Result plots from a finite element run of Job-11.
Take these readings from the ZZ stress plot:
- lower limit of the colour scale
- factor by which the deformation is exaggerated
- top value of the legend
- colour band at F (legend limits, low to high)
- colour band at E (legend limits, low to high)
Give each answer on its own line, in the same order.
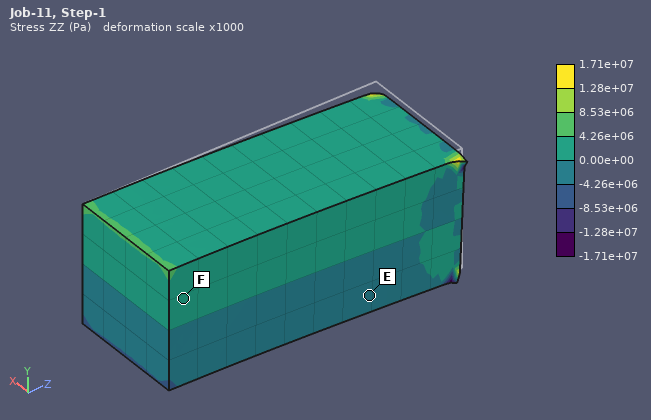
-1.71e+07 Pa
1000
1.71e+07 Pa
0.00e+00 to 4.26e+06 Pa
-4.26e+06 to 0.00e+00 Pa
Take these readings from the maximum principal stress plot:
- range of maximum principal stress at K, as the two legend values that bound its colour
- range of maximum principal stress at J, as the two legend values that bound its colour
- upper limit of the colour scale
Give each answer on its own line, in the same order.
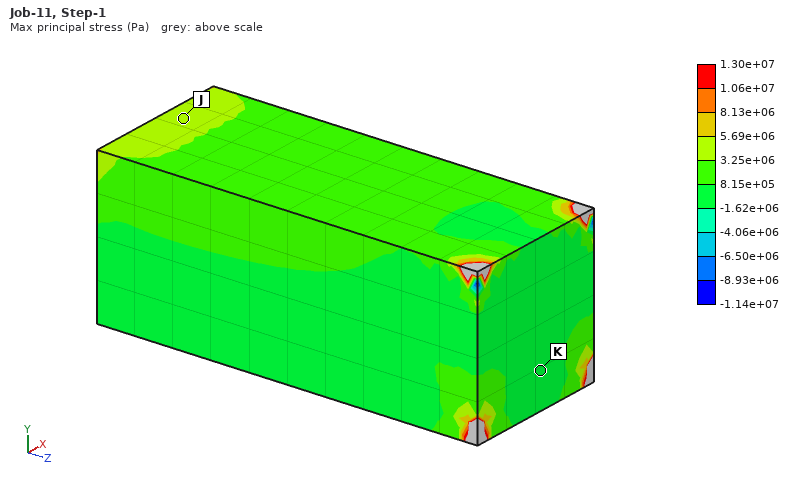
-1.62e+06 to 8.15e+05 Pa
3.25e+06 to 5.69e+06 Pa
1.30e+07 Pa
